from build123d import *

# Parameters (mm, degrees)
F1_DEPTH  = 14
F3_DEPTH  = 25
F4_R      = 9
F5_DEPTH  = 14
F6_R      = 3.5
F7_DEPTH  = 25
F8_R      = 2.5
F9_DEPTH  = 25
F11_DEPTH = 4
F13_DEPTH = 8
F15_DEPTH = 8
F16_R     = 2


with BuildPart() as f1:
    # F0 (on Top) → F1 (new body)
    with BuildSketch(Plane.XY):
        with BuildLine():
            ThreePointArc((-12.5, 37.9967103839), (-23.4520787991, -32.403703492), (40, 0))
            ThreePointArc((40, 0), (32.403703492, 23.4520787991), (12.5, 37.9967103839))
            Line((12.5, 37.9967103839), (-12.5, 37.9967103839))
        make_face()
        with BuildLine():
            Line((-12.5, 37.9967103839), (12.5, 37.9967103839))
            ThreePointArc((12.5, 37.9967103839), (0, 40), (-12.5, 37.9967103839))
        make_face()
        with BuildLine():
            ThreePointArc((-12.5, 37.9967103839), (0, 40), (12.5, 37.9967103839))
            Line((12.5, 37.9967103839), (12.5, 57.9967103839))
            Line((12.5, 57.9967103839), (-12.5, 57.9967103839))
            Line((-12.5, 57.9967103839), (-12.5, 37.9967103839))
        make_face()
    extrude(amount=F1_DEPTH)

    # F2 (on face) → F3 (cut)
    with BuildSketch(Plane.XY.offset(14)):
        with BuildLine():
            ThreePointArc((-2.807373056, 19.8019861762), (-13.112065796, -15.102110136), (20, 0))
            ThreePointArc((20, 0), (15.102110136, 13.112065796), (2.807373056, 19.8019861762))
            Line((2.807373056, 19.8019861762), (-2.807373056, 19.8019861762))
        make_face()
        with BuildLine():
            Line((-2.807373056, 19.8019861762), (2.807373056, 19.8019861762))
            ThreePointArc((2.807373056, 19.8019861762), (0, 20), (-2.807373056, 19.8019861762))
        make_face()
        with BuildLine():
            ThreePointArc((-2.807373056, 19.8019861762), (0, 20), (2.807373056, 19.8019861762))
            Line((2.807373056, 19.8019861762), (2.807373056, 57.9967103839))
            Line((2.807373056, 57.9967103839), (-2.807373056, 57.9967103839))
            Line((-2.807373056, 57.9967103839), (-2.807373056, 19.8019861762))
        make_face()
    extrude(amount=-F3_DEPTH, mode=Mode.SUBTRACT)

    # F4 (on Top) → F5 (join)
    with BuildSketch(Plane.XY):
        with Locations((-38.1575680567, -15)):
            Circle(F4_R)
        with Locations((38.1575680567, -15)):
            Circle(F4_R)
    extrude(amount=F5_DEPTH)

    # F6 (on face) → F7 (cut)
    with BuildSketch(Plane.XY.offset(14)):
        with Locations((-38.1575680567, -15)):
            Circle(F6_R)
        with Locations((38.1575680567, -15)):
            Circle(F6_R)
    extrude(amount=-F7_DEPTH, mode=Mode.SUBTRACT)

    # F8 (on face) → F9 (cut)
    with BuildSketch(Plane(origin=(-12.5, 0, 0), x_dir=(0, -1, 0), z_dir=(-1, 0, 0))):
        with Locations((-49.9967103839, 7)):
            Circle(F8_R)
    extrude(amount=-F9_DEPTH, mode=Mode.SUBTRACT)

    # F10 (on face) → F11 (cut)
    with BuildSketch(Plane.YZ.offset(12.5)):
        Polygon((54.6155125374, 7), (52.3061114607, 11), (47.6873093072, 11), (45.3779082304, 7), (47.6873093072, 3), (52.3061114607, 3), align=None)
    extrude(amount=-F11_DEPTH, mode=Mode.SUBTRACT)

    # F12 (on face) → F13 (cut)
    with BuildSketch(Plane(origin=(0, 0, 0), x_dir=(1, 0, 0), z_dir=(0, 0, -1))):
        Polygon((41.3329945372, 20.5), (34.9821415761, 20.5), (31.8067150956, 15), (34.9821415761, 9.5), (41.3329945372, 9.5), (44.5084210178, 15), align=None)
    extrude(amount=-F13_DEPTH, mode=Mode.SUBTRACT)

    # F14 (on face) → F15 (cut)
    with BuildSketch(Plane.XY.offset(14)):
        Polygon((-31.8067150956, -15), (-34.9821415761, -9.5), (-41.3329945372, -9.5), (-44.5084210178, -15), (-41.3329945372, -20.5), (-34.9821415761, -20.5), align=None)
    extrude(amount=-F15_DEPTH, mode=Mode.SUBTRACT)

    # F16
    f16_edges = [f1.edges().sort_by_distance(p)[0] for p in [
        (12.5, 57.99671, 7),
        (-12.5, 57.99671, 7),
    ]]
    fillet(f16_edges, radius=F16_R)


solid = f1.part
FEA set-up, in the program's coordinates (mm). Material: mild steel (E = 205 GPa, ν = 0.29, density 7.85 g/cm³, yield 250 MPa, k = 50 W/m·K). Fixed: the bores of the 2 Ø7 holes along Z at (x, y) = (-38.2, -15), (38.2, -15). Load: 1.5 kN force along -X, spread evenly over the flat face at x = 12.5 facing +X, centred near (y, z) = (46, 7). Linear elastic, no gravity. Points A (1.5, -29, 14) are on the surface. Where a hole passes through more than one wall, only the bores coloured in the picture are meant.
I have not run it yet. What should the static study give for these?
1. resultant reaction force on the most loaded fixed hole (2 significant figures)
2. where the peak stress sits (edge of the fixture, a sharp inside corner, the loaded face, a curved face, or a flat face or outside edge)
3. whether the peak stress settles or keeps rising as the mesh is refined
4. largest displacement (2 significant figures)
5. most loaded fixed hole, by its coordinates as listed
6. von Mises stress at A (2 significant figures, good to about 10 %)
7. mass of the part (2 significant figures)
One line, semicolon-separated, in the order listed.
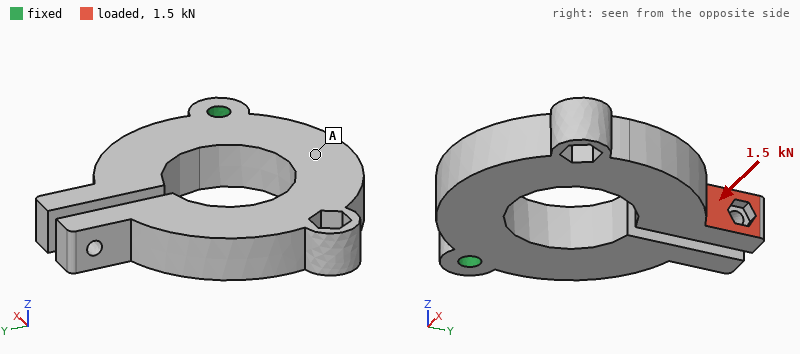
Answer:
3.0 kN; edge of the fixture; keeps rising; 0.13 mm; (38.2, -15); 13 MPa; 450 g
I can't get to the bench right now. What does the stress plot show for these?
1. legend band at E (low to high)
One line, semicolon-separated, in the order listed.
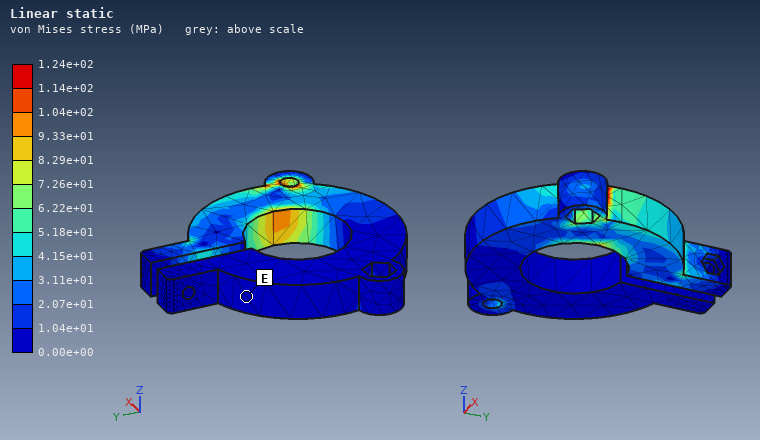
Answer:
0.00e+00 to 1.04e+01 MPa
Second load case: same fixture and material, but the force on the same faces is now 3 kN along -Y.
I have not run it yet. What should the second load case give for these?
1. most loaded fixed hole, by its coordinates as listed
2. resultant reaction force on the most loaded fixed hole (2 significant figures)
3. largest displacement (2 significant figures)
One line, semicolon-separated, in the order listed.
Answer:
(38.2, -15); 2.5 kN; 70 µm
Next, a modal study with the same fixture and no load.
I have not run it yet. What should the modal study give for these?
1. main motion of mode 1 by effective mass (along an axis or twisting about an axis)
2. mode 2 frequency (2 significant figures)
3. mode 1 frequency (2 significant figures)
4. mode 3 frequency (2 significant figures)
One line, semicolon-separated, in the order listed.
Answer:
along Z; 1800 Hz; 1500 Hz; 2700 Hz
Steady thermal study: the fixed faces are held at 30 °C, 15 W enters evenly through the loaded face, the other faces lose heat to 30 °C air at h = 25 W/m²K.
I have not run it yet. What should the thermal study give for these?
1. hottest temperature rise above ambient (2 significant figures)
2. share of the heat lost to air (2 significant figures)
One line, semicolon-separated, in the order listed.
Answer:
78 K; 34 %
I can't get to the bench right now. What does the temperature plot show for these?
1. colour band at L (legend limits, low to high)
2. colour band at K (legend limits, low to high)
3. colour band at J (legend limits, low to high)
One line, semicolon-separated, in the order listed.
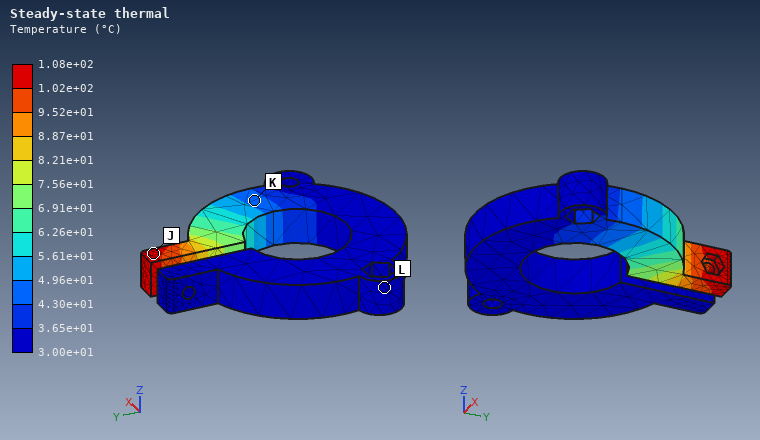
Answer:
3.00e+01 to 3.65e+01 °C; 4.30e+01 to 4.96e+01 °C; 1.02e+02 to 1.08e+02 °C
